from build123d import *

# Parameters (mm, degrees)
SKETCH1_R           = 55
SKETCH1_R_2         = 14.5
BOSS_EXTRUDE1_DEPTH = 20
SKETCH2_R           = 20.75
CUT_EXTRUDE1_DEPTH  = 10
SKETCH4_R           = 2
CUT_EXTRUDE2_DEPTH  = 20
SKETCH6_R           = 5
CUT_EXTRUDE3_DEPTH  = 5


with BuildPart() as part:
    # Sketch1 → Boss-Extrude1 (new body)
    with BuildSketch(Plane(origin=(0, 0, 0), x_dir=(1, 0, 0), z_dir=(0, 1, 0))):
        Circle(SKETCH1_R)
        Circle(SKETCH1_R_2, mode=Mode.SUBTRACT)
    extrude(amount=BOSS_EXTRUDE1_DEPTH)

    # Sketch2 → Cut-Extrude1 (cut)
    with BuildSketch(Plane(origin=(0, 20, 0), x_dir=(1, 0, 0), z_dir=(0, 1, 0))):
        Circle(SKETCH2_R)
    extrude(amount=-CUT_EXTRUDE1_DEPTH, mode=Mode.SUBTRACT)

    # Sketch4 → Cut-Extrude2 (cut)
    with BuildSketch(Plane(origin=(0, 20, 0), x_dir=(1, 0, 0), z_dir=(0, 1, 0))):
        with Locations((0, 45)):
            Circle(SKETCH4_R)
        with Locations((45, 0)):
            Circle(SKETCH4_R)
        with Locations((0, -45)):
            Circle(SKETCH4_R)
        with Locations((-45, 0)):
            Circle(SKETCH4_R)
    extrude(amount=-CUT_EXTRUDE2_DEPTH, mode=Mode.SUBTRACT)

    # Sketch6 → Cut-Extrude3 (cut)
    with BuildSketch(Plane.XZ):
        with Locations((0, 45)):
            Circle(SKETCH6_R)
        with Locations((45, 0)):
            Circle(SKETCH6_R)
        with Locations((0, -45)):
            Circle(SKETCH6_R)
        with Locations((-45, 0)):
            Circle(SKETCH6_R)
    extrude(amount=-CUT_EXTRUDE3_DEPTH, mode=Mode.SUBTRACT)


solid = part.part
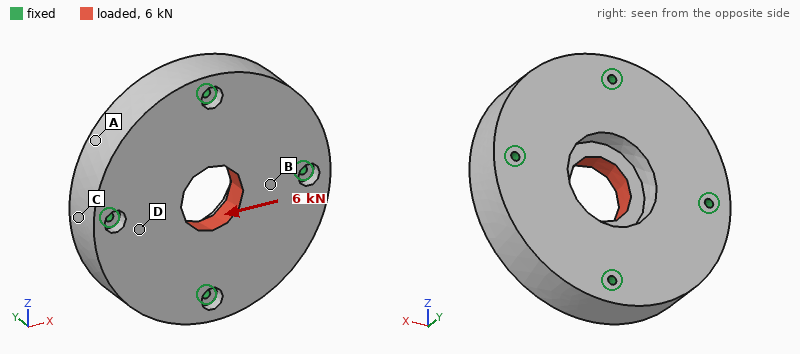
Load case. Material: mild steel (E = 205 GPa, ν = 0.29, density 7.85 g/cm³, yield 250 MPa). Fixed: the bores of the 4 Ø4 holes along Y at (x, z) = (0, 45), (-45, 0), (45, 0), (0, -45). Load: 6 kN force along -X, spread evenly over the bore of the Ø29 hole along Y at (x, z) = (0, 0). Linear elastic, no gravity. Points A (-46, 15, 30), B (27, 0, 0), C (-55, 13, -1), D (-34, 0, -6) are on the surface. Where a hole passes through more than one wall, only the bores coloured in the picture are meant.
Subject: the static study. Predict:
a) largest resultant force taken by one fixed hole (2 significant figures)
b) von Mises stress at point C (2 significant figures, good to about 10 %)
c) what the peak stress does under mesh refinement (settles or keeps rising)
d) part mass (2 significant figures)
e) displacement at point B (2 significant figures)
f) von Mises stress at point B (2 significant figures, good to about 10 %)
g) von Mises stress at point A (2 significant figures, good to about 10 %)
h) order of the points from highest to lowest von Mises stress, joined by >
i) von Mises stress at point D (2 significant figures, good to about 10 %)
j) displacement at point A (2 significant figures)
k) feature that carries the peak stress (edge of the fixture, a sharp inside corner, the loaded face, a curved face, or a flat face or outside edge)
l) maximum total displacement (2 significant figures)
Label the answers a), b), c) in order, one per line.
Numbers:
a) 1.8 kN
b) 3.5 MPa
c) keeps rising
d) 1.3 kg
e) 0.78 µm
f) 7.2 MPa
g) 1.5 MPa
h) B > D > C > A
i) 5.5 MPa
j) 0.54 µm
k) edge of the fixture
l) 1.3 µm
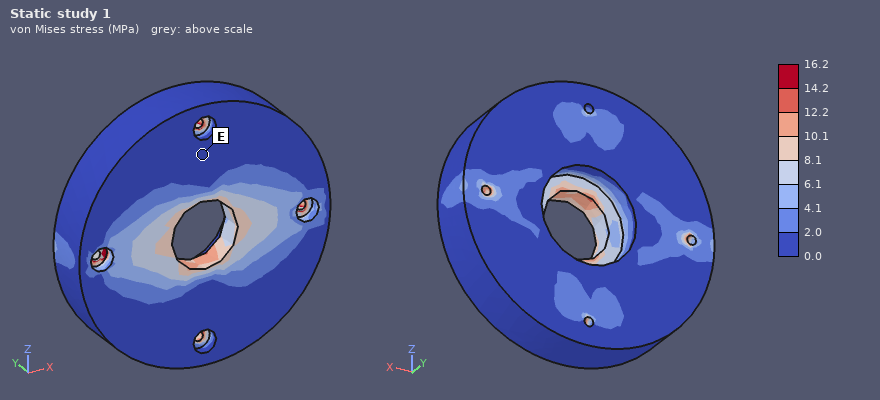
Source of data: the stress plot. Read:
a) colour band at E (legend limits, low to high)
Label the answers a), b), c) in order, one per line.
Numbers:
a) 0.0 to 2.0 MPa
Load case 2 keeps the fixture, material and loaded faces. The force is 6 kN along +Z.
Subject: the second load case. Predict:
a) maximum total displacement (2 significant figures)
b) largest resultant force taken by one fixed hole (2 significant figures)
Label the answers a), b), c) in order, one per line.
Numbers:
a) 1.3 µm
b) 1.8 kN
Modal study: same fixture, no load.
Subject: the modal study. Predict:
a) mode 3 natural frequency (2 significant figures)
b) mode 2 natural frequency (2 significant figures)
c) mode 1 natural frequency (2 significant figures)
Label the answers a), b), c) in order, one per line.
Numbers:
a) 11 kHz
b) 11 kHz
c) 10 kHz
